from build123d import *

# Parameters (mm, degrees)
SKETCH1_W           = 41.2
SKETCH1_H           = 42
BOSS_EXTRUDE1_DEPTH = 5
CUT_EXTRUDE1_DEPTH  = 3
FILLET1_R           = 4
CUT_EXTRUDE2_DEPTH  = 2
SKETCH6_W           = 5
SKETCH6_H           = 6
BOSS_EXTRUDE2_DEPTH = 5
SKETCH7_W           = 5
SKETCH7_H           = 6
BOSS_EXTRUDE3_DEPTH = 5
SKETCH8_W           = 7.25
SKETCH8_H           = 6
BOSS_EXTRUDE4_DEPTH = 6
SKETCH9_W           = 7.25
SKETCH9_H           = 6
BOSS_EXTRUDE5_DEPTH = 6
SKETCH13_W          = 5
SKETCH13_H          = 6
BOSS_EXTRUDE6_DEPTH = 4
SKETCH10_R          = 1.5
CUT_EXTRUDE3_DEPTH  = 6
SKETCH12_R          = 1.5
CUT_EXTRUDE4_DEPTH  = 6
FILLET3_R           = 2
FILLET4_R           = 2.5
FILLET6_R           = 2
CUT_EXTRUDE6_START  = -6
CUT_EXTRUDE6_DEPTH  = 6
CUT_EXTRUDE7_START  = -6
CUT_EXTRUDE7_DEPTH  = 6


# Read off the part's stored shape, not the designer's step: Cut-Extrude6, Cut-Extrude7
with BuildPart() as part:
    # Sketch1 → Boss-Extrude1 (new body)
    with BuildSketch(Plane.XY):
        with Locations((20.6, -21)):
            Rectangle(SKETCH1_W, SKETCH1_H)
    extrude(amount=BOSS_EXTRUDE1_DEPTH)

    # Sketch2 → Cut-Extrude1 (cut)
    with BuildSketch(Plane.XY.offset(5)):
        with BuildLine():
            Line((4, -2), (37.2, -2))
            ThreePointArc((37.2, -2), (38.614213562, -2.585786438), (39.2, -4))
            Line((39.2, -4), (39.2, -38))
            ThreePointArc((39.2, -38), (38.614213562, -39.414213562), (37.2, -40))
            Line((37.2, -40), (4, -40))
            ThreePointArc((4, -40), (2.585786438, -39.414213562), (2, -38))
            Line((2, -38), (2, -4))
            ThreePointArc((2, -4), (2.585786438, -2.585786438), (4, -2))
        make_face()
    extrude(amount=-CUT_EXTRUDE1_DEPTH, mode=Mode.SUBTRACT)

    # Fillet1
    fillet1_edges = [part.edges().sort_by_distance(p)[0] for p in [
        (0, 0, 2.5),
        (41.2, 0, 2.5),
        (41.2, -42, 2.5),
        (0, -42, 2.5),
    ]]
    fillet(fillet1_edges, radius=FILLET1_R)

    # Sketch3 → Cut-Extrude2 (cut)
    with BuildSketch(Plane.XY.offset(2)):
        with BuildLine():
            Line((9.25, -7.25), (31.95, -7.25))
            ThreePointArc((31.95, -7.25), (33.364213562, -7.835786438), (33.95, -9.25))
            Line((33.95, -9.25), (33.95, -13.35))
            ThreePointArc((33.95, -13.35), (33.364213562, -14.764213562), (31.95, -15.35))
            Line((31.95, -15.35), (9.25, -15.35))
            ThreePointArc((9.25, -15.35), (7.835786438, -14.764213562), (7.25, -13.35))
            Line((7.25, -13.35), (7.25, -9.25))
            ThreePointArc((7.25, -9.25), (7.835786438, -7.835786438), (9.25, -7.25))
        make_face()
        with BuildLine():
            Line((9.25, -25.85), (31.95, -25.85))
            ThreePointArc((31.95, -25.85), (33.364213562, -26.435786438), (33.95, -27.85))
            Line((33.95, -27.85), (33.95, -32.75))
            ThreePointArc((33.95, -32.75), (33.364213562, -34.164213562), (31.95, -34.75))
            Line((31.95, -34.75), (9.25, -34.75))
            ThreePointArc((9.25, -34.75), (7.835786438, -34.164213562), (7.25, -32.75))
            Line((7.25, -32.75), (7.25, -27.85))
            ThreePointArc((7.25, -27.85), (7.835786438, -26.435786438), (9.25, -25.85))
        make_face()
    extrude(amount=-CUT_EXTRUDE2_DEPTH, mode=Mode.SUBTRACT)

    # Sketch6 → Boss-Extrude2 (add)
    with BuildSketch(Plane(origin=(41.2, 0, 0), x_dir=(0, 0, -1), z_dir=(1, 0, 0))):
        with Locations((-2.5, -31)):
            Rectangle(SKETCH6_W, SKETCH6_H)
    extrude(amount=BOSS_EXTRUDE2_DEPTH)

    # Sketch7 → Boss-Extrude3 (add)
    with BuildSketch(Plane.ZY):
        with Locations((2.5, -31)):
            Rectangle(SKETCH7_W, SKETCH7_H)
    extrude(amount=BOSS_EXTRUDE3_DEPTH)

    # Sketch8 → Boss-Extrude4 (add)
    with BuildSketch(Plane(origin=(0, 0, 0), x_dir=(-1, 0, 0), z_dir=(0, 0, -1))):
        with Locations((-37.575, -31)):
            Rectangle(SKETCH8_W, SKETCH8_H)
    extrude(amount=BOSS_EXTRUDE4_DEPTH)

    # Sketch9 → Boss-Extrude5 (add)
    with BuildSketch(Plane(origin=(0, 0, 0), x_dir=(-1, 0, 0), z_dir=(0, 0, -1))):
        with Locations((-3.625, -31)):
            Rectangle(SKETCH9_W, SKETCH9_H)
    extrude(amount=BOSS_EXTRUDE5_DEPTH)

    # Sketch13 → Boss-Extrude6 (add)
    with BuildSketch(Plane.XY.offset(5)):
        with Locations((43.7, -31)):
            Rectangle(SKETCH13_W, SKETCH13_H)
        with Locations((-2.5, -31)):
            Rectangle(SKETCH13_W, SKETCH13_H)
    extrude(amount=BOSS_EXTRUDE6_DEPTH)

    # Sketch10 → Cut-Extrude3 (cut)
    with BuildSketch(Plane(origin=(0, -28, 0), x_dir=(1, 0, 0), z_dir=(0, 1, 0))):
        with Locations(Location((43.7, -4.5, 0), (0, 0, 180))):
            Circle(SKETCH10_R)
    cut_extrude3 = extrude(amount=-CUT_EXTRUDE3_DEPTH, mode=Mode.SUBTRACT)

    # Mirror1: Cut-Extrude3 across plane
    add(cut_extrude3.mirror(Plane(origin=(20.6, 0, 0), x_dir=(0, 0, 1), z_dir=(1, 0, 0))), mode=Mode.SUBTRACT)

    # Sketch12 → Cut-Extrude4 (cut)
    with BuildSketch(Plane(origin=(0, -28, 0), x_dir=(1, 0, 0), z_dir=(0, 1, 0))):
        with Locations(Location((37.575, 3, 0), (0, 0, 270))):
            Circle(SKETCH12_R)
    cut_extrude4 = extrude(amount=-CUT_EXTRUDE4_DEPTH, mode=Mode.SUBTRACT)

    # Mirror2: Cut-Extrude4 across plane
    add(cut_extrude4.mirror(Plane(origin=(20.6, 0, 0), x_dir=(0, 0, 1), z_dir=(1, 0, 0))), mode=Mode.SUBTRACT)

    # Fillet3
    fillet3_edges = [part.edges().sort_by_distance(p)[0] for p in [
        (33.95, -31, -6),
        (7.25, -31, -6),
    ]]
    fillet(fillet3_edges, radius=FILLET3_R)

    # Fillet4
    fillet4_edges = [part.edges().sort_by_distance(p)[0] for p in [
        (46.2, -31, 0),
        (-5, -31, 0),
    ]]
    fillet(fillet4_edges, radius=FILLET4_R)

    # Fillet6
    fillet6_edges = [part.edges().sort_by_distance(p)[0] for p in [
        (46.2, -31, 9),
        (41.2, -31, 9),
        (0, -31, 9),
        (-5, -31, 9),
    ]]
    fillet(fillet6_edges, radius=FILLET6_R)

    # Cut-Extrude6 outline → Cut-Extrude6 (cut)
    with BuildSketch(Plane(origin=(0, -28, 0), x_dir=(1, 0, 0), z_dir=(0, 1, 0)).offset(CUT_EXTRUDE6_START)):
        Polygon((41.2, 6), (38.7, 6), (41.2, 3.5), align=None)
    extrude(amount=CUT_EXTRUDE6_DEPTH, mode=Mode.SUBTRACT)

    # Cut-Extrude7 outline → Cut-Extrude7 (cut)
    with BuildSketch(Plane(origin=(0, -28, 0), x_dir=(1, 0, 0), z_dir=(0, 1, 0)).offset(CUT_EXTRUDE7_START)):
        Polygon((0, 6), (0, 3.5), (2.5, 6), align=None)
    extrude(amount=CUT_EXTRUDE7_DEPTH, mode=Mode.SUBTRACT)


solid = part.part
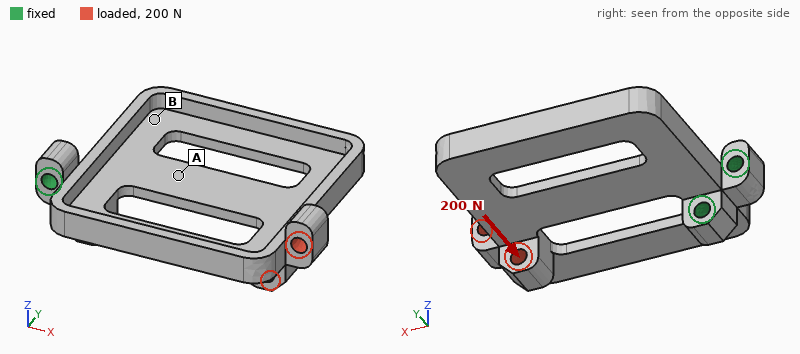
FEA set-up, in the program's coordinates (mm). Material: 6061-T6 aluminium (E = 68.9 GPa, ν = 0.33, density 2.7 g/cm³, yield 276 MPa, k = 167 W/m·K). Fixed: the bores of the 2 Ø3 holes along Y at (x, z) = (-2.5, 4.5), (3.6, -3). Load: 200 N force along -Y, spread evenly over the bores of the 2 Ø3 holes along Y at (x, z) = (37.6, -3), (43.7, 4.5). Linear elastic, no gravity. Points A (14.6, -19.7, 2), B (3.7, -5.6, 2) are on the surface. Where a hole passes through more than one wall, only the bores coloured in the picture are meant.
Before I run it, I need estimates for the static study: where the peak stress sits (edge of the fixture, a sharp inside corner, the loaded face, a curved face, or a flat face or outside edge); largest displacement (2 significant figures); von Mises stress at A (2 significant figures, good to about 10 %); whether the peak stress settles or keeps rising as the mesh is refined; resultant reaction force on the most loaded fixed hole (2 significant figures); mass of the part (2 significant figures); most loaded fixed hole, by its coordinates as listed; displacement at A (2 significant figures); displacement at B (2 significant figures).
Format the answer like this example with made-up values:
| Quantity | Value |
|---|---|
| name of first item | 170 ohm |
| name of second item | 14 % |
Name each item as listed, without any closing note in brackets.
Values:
| Quantity | Value |
|---|---|
| where the peak stress sits | a sharp inside corner |
| largest displacement | 0.26 mm |
| von Mises stress at A | 24 MPa |
| whether the peak stress settles or keeps rising as the mesh is refined | keeps rising |
| resultant reaction force on the most loaded fixed hole | 700 N |
| mass of the part | 12 g |
| most loaded fixed hole, by its coordinates as listed | (3.6, -3) |
| displacement at A | 0.082 mm |
| displacement at B | 0.13 mm |
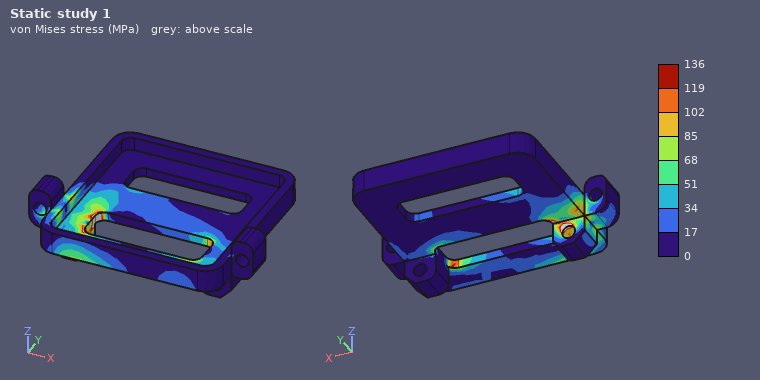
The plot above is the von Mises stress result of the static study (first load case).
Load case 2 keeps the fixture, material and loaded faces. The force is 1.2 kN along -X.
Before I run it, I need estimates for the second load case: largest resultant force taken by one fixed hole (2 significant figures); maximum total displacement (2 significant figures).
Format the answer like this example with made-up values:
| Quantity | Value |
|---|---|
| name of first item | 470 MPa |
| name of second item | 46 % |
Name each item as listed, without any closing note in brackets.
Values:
| Quantity | Value |
|---|---|
| largest resultant force taken by one fixed hole | 660 N |
| maximum total displacement | 0.16 mm |
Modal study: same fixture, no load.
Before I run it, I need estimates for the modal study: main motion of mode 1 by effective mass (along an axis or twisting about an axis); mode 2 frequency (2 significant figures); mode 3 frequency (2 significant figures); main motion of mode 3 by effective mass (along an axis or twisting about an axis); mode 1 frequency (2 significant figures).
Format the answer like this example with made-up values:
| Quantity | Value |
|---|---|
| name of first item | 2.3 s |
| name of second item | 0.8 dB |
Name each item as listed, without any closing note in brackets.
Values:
| Quantity | Value |
|---|---|
| main motion of mode 1 by effective mass | along Z |
| mode 2 frequency | 1500 Hz |
| mode 3 frequency | 2200 Hz |
| main motion of mode 3 by effective mass | along Y |
| mode 1 frequency | 760 Hz |
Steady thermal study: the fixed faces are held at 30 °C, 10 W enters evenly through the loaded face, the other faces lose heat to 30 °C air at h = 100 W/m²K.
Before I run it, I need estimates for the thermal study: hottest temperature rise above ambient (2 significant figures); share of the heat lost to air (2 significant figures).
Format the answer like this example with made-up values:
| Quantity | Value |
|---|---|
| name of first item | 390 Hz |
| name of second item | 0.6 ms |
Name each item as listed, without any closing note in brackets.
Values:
| Quantity | Value |
|---|---|
| hottest temperature rise above ambient | 36 K |
| share of the heat lost to air | 60 % |
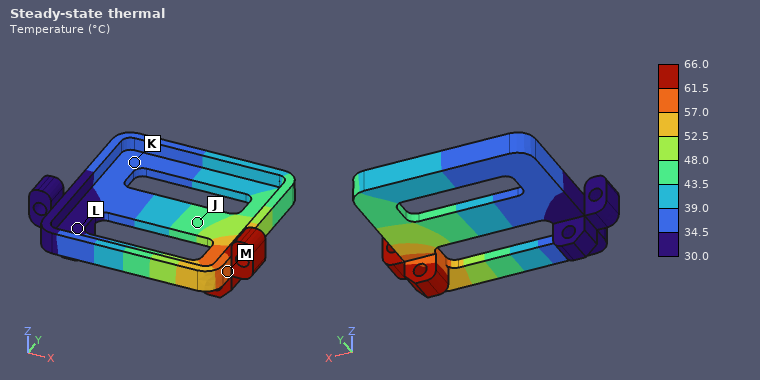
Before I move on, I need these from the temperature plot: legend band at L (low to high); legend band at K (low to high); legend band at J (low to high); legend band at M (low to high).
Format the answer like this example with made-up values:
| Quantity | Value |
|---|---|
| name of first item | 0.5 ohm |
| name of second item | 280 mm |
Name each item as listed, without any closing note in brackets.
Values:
| Quantity | Value |
|---|---|
| legend band at L | 30.0 to 34.5 °C |
| legend band at K | 34.5 to 39.0 °C |
| legend band at J | 43.5 to 48.0 °C |
| legend band at M | 57.0 to 61.5 °C |
